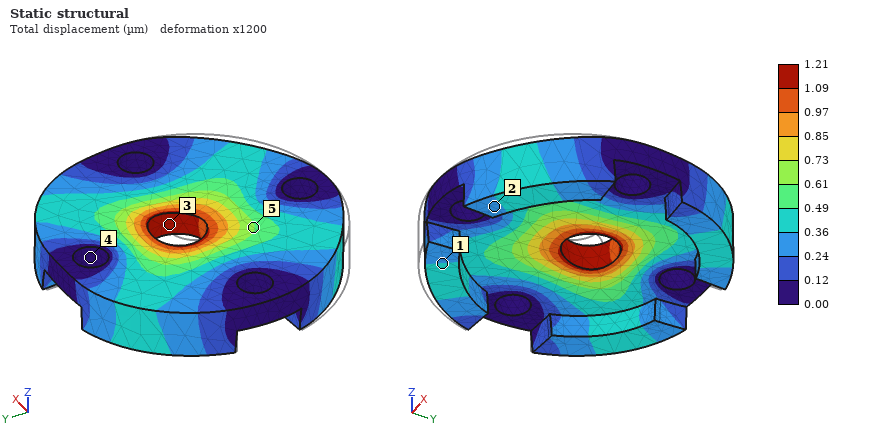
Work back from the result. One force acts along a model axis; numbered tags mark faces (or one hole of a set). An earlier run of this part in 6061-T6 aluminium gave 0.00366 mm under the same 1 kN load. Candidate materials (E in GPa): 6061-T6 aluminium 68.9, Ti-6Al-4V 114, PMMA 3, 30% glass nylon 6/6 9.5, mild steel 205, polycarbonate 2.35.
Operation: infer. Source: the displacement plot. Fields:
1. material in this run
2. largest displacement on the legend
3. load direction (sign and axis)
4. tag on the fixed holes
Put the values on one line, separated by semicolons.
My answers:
mild steel; 1.21 µm; +Y; 4
